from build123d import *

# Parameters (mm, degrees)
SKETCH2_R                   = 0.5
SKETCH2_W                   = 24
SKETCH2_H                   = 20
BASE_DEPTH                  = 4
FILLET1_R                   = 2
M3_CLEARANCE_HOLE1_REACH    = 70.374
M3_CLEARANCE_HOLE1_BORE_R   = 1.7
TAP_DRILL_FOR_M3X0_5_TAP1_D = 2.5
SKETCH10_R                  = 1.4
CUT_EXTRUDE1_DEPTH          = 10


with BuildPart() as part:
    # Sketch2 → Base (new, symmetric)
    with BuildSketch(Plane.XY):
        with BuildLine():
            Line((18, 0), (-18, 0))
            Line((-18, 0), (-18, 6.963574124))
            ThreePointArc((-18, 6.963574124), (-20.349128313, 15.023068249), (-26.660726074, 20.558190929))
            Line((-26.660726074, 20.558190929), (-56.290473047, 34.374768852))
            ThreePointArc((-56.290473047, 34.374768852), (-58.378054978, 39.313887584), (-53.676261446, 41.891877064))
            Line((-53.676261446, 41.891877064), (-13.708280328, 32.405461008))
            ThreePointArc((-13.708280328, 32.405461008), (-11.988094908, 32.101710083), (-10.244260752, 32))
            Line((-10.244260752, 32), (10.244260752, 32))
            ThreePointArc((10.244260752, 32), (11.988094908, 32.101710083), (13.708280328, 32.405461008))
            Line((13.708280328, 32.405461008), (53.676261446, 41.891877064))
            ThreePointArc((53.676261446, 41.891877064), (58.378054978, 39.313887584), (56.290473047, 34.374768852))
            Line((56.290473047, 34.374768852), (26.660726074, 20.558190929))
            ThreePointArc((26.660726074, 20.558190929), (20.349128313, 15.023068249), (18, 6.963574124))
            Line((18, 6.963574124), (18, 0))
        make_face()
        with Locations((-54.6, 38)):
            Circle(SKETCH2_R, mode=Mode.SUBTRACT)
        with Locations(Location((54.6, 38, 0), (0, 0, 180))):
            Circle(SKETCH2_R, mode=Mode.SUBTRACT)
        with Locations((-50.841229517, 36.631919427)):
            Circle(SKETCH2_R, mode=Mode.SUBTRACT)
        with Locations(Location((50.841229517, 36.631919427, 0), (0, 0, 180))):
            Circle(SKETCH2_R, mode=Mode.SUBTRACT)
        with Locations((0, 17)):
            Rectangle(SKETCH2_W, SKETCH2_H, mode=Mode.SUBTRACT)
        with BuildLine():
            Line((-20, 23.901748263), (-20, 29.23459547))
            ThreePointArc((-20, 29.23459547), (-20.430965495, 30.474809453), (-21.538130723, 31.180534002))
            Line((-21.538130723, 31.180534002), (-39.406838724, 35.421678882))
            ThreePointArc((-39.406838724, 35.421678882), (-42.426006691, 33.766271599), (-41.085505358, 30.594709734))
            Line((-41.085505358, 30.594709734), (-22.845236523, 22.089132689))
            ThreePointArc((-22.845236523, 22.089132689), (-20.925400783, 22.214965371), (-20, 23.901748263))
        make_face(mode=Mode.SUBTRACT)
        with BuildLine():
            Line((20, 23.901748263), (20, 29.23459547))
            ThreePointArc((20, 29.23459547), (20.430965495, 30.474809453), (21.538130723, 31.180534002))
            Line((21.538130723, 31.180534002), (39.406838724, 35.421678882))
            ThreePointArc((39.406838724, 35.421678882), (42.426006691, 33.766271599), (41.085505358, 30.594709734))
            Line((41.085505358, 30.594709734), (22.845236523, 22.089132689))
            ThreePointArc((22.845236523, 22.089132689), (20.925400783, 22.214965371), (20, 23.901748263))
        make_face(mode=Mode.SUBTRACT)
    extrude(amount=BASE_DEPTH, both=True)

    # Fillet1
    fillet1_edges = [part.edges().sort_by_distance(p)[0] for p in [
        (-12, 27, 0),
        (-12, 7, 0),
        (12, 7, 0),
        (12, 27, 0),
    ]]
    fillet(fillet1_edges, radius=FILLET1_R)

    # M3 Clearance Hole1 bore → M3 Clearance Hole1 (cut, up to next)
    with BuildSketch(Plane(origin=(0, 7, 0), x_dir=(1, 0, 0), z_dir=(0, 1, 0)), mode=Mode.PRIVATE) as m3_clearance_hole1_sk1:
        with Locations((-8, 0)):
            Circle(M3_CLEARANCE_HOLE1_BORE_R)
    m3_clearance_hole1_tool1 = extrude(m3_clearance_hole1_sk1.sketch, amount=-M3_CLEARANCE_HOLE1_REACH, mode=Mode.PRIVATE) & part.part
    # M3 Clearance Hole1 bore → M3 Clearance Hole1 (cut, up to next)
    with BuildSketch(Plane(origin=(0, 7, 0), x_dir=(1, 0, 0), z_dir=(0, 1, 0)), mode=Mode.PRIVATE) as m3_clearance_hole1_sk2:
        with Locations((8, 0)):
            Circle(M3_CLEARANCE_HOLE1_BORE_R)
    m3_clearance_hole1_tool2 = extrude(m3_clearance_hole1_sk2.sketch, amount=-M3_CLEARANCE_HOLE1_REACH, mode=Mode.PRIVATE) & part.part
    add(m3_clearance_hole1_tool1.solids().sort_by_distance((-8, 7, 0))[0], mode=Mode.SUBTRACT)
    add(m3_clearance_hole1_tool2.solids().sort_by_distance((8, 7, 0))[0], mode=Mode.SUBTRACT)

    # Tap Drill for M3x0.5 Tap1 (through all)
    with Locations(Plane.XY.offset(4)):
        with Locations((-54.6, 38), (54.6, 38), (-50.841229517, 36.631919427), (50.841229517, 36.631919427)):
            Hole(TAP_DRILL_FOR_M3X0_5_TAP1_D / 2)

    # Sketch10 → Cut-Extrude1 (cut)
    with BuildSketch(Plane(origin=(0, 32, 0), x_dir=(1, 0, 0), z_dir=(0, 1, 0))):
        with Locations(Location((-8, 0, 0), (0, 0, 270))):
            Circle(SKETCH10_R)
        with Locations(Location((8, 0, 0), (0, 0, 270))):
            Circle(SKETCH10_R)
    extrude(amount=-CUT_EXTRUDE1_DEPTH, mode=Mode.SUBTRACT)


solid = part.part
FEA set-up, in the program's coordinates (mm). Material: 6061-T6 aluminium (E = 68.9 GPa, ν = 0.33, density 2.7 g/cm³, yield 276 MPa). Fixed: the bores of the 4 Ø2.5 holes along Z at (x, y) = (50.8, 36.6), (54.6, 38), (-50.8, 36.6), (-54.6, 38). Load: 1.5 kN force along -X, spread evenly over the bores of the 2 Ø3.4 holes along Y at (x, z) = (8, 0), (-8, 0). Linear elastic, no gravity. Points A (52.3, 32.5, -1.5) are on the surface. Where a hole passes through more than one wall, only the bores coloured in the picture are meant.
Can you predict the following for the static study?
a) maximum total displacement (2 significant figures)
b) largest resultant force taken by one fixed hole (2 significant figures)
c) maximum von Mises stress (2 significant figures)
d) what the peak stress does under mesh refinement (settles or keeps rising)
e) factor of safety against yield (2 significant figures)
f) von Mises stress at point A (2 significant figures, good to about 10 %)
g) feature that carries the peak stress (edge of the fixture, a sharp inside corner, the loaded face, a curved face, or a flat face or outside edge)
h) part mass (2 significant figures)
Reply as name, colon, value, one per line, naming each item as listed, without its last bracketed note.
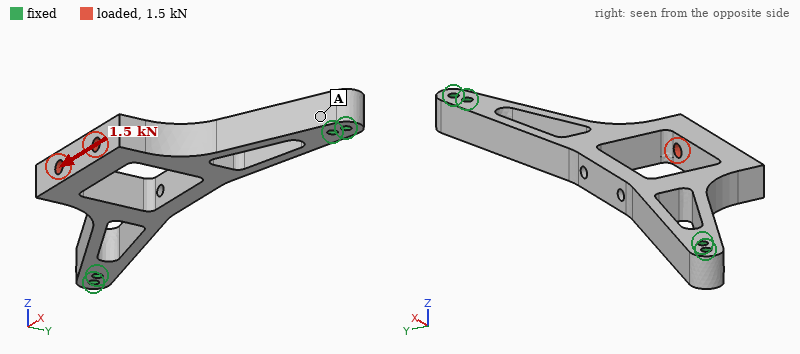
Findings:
maximum total displacement: 63 µm
largest resultant force taken by one fixed hole: 700 N
maximum von Mises stress: 160 MPa
what the peak stress does under mesh refinement: settles
factor of safety against yield: 1.7
von Mises stress at point A: 19 MPa
feature that carries the peak stress: the loaded face
part mass: 29 g
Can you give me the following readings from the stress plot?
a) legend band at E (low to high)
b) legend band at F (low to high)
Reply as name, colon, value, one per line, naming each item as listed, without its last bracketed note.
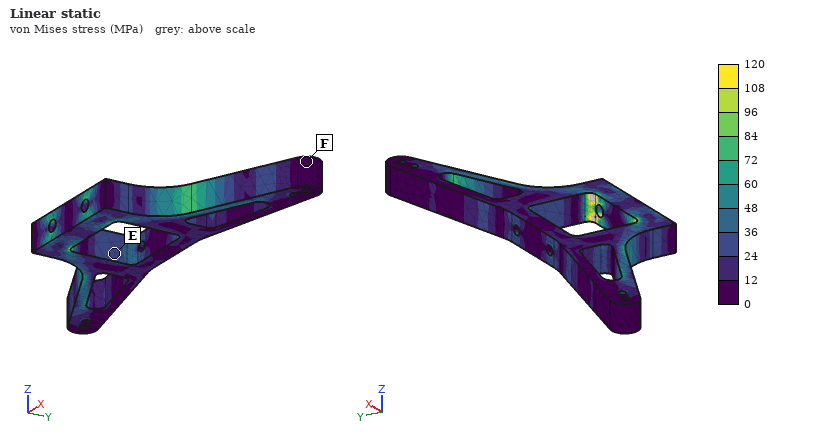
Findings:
legend band at E: 24 to 36 MPa
legend band at F: 0 to 12 MPa
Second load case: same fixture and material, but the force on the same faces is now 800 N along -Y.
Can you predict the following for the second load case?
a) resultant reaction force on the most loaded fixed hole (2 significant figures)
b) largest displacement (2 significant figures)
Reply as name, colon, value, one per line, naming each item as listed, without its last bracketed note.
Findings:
resultant reaction force on the most loaded fixed hole: 760 N
largest displacement: 43 µm
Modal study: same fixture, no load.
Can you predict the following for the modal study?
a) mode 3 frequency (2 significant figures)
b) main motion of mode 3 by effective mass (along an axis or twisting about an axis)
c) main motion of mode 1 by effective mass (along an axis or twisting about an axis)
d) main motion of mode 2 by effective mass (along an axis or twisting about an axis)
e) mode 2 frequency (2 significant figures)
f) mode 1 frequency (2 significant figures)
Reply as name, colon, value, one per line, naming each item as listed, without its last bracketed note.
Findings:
mode 3 frequency: 4900 Hz
main motion of mode 3 by effective mass: along Y
main motion of mode 1 by effective mass: along Z
main motion of mode 2 by effective mass: along Z
mode 2 frequency: 4600 Hz
mode 1 frequency: 1500 Hz
